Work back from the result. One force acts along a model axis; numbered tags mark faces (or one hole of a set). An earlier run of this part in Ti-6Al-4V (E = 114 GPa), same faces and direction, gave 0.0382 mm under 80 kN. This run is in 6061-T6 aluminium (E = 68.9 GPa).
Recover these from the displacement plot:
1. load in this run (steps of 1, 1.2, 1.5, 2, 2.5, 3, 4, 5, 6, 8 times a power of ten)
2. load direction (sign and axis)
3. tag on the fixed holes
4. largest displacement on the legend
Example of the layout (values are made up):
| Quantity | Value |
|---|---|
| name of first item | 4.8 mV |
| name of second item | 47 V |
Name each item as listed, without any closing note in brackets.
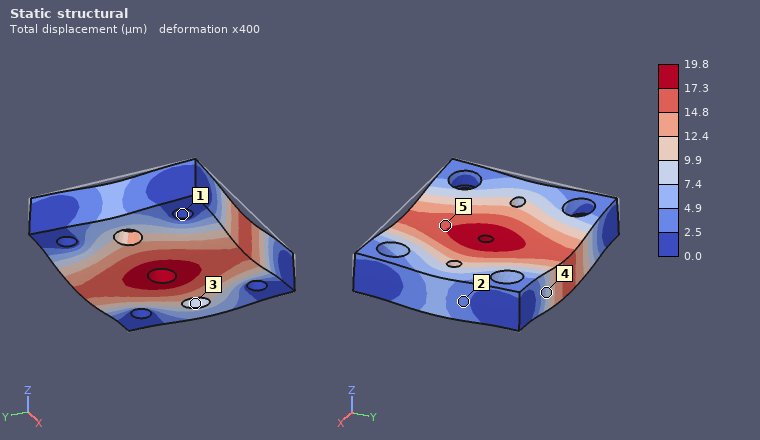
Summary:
| Quantity | Value |
|---|---|
| load in this run | 25 kN |
| load direction | -Z |
| tag on the fixed holes | 1 |
| largest displacement on the legend | 19.8 µm |
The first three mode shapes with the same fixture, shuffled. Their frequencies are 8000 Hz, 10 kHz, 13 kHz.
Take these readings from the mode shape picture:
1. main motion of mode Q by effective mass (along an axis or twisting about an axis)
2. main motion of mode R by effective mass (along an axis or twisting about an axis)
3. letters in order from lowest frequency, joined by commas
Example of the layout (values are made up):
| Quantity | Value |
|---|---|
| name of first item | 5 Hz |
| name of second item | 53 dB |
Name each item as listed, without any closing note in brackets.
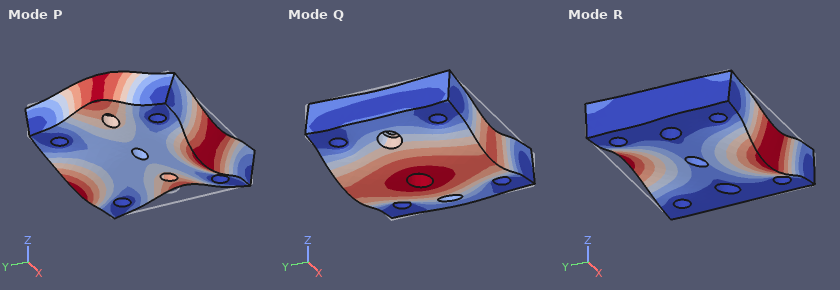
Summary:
| Quantity | Value |
|---|---|
| main motion of mode Q by effective mass | along Z |
| main motion of mode R by effective mass | twisting about X |
| letters in order from lowest frequency, joined by commas | Q, R, P |
